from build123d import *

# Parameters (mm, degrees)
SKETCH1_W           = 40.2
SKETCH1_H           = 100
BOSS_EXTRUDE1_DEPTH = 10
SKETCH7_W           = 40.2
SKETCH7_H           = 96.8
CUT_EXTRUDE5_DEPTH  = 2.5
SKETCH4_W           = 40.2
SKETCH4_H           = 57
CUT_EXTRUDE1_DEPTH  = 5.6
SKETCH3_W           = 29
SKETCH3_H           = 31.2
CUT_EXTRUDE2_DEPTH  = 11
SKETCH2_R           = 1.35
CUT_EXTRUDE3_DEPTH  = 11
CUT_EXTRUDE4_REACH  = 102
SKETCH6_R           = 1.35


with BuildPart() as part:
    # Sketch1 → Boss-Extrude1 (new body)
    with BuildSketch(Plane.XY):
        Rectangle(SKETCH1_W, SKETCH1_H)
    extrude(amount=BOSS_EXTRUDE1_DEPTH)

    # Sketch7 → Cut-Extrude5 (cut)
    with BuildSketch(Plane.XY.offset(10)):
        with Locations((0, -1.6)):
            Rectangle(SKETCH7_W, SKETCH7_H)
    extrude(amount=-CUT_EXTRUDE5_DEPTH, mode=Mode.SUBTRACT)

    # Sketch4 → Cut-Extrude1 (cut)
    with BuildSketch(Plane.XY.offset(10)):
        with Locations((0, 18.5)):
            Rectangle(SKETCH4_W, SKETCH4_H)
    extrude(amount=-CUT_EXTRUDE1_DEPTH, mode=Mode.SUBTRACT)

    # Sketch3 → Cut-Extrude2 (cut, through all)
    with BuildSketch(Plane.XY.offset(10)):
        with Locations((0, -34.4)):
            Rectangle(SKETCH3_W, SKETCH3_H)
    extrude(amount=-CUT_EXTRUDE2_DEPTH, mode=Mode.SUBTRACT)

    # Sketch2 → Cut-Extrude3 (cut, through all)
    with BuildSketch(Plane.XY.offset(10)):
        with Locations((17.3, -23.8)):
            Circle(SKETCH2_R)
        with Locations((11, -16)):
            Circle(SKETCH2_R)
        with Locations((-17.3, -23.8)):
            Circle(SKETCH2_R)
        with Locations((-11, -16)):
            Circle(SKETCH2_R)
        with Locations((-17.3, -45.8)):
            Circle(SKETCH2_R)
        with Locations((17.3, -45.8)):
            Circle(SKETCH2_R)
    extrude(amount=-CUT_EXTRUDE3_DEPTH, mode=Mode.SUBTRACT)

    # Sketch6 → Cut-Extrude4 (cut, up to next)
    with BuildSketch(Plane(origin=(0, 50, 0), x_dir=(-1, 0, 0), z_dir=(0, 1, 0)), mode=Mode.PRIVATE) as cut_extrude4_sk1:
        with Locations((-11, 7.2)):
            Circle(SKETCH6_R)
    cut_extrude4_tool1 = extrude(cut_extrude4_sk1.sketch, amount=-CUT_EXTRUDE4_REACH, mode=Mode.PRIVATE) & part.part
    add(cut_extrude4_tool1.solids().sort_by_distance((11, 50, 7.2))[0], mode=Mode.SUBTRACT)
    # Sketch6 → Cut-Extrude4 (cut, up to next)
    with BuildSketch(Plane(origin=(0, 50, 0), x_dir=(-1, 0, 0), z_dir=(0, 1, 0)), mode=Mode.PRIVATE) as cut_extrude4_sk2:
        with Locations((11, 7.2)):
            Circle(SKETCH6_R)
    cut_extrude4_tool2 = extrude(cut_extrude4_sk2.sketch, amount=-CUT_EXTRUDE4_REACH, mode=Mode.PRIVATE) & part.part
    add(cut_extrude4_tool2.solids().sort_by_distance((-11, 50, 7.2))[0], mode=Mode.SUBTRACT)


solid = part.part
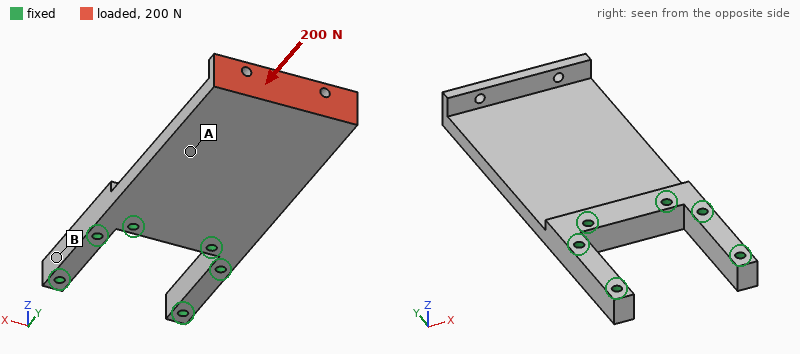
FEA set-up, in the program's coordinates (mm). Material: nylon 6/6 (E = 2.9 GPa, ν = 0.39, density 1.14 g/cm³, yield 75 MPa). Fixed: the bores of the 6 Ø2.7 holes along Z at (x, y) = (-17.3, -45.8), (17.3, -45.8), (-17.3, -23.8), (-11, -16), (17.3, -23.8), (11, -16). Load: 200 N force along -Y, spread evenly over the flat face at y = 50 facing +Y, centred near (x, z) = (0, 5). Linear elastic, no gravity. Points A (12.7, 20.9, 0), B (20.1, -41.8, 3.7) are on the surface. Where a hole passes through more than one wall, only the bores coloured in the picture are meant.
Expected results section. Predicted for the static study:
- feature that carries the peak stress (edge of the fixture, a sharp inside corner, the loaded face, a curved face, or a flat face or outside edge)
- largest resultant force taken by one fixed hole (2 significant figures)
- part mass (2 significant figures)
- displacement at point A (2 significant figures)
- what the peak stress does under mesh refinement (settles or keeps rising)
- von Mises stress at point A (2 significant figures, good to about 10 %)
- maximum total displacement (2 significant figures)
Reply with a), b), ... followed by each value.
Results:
a) edge of the fixture
b) 79 N
c) 19 g
d) 0.34 mm
e) keeps rising
f) 3.0 MPa
g) 1.3 mm
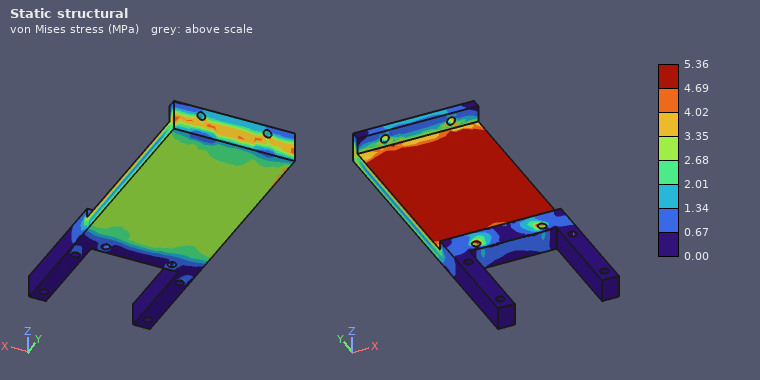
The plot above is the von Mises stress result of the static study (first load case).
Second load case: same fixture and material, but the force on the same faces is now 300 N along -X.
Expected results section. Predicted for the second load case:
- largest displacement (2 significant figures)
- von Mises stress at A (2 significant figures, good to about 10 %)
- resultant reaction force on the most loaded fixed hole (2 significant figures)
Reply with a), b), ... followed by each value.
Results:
a) 1.2 mm
b) 5.6 MPa
c) 450 N
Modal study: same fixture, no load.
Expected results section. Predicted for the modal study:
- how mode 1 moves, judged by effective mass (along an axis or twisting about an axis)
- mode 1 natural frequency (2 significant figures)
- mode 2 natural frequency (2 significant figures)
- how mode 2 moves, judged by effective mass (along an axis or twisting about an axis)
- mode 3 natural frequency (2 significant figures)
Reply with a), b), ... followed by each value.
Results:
a) along Z
b) 260 Hz
c) 880 Hz
d) twisting about Y
e) 1600 Hz
